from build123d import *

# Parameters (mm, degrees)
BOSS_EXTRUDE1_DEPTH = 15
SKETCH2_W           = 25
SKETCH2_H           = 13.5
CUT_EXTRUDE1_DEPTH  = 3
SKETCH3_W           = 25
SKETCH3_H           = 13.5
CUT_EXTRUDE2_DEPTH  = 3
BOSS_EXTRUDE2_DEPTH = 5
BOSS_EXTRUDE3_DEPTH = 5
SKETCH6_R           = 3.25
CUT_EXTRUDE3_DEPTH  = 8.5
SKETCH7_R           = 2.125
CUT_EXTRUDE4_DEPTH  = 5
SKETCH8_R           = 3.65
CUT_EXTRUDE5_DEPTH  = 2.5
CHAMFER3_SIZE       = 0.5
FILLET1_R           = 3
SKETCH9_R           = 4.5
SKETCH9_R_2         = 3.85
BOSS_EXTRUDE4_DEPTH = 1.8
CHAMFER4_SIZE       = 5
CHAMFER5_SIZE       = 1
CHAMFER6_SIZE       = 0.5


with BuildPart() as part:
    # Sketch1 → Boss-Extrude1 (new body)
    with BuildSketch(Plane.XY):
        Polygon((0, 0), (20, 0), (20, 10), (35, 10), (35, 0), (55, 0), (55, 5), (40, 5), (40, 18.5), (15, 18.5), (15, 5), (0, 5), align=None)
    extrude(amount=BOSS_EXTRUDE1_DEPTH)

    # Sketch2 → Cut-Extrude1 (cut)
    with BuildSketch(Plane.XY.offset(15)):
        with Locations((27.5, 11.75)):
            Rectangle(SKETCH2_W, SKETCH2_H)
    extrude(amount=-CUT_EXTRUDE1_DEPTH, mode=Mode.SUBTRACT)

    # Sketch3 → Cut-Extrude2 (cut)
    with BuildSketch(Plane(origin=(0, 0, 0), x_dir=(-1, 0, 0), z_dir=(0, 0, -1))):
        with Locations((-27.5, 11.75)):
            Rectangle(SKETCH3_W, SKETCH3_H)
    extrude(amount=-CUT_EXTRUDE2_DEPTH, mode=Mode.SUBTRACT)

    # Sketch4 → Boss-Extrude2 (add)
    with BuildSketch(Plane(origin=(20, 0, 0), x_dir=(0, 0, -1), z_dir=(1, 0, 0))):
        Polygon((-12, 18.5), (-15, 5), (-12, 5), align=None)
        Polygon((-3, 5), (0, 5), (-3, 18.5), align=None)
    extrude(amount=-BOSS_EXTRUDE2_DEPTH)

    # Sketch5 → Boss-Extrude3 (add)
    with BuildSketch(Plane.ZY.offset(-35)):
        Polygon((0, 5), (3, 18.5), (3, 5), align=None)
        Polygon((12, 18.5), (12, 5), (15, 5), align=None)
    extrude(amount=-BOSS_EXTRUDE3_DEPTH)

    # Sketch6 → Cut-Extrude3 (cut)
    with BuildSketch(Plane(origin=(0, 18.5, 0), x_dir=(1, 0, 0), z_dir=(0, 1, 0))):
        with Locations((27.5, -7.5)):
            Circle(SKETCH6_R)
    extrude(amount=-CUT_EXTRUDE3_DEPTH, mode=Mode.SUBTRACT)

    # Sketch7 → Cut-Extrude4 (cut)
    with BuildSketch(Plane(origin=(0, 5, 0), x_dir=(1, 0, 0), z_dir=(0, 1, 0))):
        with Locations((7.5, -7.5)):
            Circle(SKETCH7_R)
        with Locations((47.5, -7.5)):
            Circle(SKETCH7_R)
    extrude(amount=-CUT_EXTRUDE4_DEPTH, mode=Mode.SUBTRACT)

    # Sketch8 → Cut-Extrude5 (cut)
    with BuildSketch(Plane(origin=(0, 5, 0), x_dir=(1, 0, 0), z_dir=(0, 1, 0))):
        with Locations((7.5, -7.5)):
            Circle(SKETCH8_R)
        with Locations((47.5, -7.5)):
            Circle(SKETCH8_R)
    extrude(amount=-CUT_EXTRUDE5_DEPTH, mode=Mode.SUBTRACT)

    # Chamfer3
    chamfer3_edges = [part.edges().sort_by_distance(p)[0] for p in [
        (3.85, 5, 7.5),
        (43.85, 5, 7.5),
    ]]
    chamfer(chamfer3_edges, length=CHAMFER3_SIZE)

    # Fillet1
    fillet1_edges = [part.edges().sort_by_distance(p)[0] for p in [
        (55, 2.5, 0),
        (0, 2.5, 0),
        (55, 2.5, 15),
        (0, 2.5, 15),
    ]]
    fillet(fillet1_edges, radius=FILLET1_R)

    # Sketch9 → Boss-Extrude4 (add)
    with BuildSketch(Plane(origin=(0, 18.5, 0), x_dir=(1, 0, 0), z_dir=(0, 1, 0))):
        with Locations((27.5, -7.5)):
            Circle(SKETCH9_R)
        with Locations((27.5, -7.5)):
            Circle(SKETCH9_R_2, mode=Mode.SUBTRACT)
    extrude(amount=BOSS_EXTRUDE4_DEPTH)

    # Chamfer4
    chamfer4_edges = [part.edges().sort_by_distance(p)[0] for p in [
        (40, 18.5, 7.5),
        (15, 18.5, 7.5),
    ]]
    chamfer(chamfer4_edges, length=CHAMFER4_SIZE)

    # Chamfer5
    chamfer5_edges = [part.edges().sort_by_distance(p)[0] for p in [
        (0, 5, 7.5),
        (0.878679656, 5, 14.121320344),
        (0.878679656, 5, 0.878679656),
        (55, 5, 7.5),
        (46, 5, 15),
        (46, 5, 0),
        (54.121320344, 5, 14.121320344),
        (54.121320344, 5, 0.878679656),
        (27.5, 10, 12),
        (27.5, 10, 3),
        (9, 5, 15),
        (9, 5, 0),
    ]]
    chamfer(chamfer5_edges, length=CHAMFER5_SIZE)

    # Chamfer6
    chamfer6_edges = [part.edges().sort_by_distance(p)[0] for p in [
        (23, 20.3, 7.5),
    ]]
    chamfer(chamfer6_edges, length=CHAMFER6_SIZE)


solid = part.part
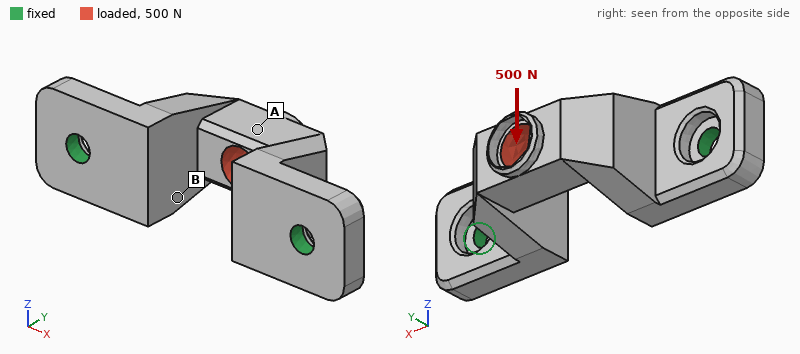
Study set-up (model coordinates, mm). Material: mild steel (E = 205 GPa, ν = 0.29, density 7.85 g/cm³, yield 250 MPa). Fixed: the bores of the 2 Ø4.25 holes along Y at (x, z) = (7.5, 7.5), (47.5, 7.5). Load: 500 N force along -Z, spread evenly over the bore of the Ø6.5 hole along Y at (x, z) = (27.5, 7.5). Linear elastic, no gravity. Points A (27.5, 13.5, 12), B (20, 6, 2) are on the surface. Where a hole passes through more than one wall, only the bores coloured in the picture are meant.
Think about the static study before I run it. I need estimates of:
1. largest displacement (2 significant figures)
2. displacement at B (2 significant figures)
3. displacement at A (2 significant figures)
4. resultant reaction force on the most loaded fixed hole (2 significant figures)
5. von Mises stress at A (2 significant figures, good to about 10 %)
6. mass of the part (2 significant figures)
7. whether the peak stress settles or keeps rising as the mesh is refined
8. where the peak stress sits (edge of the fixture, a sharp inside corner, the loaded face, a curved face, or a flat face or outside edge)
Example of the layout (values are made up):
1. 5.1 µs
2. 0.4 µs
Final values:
1. 25 µm
2. 9.7 µm
3. 17 µm
4. 250 N
5. 25 MPa
6. 38 g
7. keeps rising
8. edge of the fixture
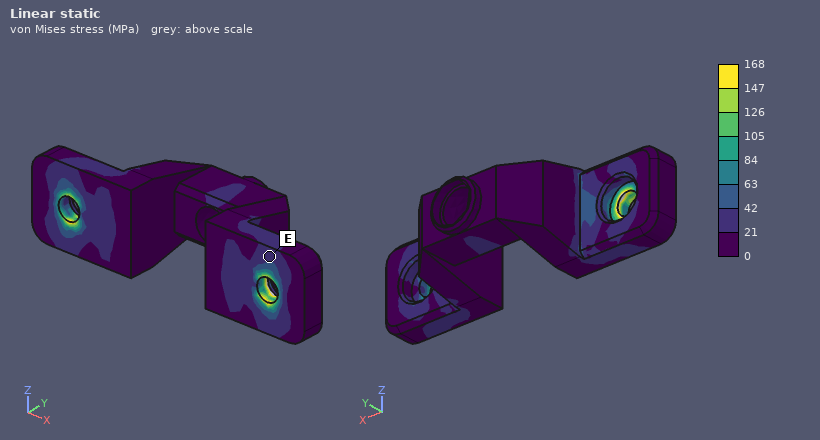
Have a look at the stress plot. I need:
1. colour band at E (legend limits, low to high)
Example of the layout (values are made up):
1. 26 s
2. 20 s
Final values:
1. 21 to 42 MPa
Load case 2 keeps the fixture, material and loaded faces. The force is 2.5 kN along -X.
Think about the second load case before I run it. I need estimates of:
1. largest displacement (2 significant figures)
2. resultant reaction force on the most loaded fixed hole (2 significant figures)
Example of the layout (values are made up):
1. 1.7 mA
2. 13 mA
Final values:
1. 12 µm
2. 1.5 kN
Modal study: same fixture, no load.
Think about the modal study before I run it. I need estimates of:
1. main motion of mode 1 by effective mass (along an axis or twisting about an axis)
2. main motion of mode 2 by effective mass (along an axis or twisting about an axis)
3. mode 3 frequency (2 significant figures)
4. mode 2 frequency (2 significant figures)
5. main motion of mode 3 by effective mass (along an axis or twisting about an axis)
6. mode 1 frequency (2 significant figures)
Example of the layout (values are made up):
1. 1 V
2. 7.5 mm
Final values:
1. along Z
2. along Y
3. 17 kHz
4. 16 kHz
5. along X
6. 7000 Hz
